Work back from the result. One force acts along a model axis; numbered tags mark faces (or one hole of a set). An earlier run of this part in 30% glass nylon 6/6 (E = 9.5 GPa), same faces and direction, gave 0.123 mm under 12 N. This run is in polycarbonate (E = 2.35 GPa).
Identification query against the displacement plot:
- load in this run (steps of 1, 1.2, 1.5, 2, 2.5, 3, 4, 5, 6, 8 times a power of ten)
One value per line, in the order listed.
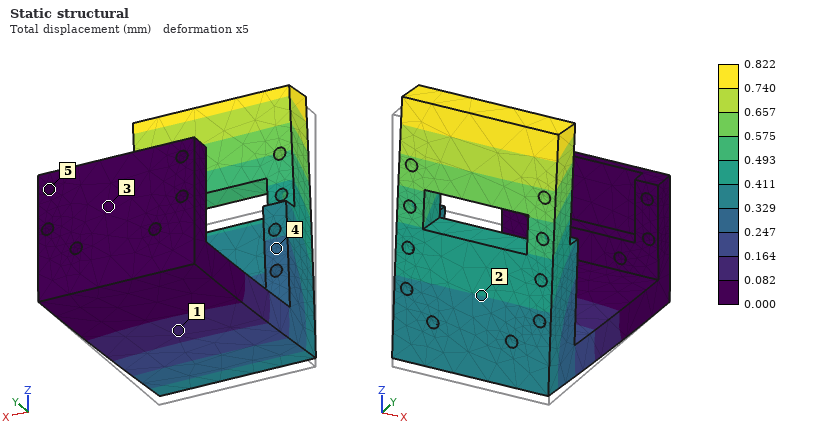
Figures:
20 N
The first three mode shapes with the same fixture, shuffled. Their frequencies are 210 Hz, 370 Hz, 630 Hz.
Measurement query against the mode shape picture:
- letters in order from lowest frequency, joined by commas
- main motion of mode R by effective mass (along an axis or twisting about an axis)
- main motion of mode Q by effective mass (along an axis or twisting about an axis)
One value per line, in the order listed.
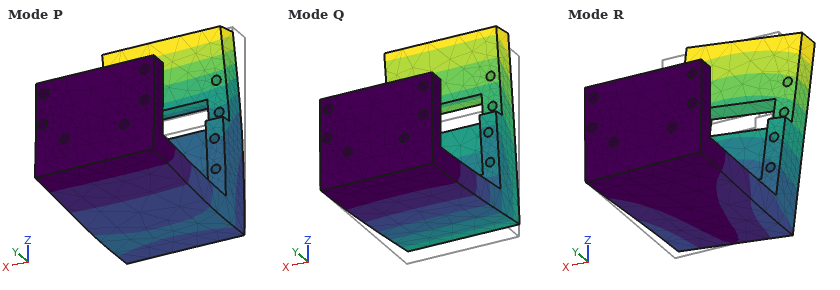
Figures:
Q, R, P
along X
along Z
